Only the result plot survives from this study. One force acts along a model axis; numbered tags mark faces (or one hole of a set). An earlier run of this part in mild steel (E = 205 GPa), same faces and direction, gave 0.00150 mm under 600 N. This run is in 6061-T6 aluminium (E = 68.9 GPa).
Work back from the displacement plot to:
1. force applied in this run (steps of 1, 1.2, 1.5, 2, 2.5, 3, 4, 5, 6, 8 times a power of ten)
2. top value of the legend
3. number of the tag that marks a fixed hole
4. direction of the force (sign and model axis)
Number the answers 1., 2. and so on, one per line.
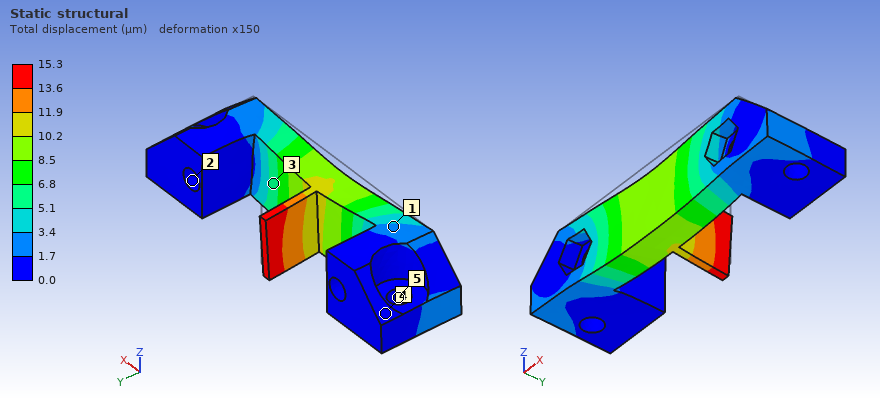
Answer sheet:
1. 2 kN
2. 15.3 µm
3. 2
4. -Z
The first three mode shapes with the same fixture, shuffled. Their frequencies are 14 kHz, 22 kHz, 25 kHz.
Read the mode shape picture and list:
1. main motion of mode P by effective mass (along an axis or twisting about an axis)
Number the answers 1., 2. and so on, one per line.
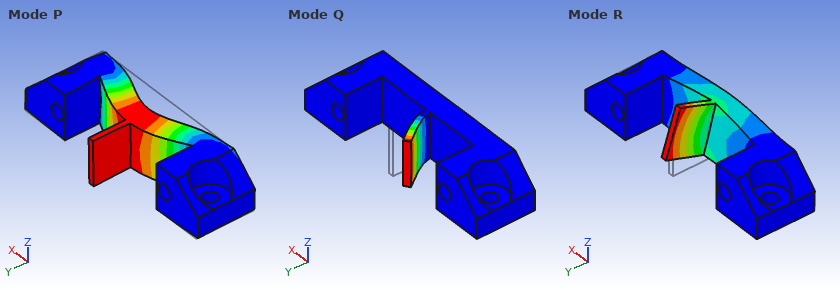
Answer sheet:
1. along Y
